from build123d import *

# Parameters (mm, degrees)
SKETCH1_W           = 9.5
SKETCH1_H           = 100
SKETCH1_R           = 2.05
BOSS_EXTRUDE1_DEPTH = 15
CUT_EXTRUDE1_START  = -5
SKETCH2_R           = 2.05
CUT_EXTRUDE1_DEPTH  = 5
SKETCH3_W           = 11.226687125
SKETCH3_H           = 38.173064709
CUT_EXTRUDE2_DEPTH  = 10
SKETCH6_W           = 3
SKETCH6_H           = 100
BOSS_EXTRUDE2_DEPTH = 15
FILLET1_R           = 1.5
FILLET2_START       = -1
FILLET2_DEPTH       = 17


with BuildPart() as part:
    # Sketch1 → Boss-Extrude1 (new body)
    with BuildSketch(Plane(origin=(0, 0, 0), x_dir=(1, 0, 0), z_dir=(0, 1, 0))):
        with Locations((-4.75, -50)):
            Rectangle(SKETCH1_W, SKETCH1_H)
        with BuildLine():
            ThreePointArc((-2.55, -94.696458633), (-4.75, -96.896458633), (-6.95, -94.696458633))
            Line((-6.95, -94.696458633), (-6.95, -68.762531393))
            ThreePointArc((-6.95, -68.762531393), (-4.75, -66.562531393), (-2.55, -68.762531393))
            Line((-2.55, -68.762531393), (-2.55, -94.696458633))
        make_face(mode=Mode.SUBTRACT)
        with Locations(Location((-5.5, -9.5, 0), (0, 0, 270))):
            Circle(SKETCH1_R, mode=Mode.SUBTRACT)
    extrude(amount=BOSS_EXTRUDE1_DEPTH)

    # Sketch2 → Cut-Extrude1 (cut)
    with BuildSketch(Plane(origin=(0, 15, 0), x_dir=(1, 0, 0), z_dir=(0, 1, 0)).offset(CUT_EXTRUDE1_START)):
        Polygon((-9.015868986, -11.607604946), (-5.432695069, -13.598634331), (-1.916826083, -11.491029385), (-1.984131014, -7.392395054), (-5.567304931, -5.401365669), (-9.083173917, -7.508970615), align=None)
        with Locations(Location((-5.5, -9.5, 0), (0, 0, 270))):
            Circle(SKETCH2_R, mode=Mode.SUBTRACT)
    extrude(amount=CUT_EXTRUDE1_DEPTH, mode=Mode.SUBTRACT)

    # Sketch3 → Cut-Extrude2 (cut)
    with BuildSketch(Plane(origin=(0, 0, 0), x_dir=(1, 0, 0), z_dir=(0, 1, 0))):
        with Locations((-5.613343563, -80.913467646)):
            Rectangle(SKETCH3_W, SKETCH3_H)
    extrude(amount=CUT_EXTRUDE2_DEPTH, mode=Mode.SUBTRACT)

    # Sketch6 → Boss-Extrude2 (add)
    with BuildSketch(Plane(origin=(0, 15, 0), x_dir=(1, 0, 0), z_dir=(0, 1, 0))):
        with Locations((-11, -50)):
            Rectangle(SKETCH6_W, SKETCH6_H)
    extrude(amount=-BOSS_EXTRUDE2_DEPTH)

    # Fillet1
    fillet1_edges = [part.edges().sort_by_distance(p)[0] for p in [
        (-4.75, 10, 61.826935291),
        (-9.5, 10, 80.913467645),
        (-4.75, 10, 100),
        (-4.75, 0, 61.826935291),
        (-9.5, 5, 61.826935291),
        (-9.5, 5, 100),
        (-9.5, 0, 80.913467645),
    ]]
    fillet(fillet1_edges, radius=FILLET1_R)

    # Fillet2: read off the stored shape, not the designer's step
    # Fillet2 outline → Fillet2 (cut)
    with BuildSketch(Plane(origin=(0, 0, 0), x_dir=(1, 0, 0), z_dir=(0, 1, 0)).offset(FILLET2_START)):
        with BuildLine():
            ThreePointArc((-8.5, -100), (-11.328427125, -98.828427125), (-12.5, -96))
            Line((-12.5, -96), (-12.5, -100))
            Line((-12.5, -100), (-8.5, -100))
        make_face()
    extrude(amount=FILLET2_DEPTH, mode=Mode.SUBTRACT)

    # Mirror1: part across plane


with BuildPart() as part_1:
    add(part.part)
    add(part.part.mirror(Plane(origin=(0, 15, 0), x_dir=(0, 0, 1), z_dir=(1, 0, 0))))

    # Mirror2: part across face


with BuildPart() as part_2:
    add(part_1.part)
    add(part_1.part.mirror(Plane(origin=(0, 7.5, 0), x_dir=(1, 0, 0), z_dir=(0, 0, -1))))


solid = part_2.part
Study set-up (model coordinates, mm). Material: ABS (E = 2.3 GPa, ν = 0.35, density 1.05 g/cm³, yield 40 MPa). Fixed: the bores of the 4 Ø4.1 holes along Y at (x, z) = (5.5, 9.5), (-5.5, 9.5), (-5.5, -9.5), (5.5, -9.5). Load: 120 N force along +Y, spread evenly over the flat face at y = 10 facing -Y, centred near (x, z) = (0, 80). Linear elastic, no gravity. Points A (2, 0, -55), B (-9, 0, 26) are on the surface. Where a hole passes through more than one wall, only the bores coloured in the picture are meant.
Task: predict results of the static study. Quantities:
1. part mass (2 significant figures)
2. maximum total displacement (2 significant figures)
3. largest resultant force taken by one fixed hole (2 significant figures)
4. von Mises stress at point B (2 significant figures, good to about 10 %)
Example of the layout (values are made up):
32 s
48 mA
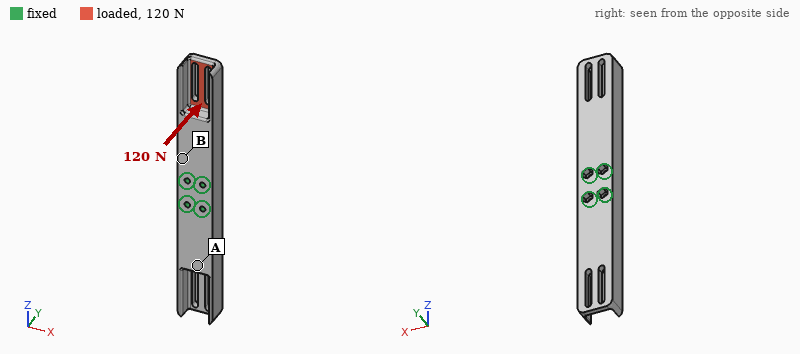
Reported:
59 g
1.7 mm
160 N
6.9 MPa
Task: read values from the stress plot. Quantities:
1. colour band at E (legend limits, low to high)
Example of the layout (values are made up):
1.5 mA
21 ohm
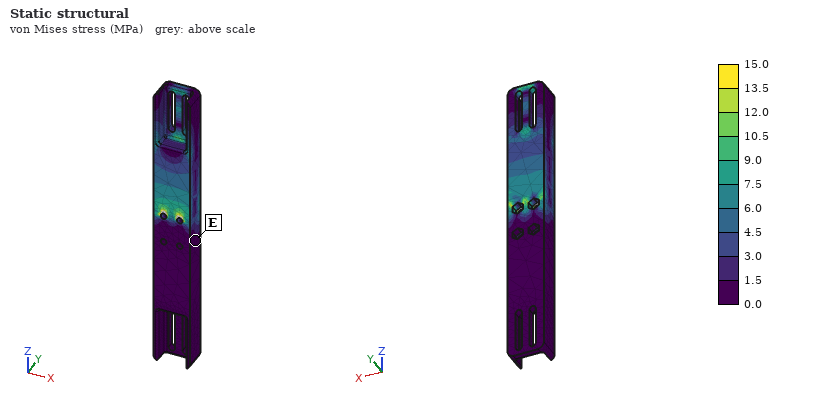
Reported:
0.0 to 1.5 MPa
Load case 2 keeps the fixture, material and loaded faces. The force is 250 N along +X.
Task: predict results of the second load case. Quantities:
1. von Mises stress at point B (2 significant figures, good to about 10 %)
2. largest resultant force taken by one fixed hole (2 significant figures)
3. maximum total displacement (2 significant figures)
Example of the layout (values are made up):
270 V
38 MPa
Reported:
6.7 MPa
950 N
2.2 mm
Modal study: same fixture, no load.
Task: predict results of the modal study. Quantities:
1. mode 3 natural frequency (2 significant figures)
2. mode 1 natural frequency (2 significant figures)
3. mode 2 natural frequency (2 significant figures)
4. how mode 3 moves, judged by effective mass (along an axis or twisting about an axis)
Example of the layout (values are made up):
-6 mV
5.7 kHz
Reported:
780 Hz
560 Hz
560 Hz
twisting about Y
